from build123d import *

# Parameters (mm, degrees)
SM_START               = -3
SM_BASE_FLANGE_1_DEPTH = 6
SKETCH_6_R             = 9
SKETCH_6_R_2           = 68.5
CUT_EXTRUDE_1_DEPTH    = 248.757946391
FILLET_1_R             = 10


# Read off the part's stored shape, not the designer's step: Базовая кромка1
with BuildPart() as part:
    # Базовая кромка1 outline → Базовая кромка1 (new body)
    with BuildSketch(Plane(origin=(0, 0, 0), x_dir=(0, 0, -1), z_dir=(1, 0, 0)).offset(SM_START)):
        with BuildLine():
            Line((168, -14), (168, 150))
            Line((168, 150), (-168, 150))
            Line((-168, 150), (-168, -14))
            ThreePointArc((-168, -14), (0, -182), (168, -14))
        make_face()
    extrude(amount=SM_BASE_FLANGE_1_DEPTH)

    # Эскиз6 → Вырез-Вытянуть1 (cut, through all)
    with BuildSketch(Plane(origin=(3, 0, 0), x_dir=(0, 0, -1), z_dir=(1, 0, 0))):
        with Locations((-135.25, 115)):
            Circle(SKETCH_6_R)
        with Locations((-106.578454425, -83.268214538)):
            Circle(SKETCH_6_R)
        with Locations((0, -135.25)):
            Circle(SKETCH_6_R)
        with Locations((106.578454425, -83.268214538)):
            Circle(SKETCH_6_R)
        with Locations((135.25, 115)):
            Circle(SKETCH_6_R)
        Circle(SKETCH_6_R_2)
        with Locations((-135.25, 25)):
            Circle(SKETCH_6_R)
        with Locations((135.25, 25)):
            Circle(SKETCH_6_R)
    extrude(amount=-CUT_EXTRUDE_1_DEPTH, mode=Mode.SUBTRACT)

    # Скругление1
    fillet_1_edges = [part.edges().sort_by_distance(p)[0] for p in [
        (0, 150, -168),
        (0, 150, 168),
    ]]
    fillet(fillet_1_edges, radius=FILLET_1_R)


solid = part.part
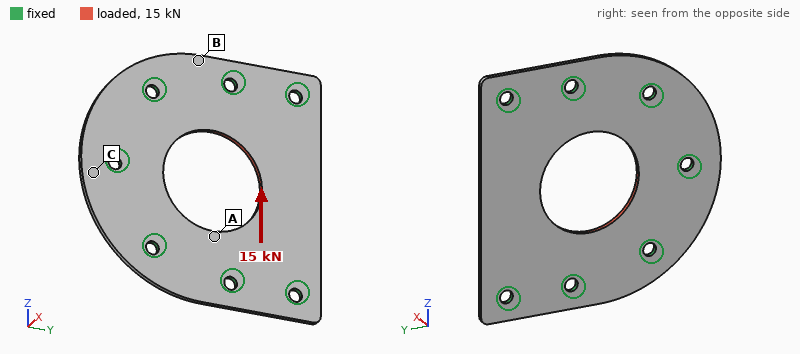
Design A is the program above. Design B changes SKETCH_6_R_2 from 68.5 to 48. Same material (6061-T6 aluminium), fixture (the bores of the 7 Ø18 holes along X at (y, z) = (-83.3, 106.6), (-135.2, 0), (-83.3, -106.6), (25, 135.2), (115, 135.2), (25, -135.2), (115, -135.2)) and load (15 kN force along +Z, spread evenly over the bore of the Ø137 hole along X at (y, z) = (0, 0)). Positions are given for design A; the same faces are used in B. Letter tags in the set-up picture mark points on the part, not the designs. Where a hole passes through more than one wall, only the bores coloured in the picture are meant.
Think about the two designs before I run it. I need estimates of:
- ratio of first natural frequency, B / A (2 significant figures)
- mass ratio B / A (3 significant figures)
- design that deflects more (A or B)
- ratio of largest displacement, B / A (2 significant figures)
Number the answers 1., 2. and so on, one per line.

1. 0.99
2. 1.09
3. B
4. 1.2
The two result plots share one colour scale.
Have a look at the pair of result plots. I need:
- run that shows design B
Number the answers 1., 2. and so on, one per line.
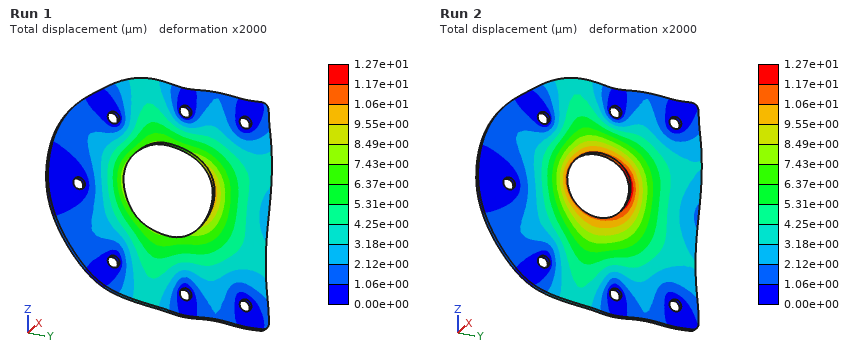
1. Run 2
